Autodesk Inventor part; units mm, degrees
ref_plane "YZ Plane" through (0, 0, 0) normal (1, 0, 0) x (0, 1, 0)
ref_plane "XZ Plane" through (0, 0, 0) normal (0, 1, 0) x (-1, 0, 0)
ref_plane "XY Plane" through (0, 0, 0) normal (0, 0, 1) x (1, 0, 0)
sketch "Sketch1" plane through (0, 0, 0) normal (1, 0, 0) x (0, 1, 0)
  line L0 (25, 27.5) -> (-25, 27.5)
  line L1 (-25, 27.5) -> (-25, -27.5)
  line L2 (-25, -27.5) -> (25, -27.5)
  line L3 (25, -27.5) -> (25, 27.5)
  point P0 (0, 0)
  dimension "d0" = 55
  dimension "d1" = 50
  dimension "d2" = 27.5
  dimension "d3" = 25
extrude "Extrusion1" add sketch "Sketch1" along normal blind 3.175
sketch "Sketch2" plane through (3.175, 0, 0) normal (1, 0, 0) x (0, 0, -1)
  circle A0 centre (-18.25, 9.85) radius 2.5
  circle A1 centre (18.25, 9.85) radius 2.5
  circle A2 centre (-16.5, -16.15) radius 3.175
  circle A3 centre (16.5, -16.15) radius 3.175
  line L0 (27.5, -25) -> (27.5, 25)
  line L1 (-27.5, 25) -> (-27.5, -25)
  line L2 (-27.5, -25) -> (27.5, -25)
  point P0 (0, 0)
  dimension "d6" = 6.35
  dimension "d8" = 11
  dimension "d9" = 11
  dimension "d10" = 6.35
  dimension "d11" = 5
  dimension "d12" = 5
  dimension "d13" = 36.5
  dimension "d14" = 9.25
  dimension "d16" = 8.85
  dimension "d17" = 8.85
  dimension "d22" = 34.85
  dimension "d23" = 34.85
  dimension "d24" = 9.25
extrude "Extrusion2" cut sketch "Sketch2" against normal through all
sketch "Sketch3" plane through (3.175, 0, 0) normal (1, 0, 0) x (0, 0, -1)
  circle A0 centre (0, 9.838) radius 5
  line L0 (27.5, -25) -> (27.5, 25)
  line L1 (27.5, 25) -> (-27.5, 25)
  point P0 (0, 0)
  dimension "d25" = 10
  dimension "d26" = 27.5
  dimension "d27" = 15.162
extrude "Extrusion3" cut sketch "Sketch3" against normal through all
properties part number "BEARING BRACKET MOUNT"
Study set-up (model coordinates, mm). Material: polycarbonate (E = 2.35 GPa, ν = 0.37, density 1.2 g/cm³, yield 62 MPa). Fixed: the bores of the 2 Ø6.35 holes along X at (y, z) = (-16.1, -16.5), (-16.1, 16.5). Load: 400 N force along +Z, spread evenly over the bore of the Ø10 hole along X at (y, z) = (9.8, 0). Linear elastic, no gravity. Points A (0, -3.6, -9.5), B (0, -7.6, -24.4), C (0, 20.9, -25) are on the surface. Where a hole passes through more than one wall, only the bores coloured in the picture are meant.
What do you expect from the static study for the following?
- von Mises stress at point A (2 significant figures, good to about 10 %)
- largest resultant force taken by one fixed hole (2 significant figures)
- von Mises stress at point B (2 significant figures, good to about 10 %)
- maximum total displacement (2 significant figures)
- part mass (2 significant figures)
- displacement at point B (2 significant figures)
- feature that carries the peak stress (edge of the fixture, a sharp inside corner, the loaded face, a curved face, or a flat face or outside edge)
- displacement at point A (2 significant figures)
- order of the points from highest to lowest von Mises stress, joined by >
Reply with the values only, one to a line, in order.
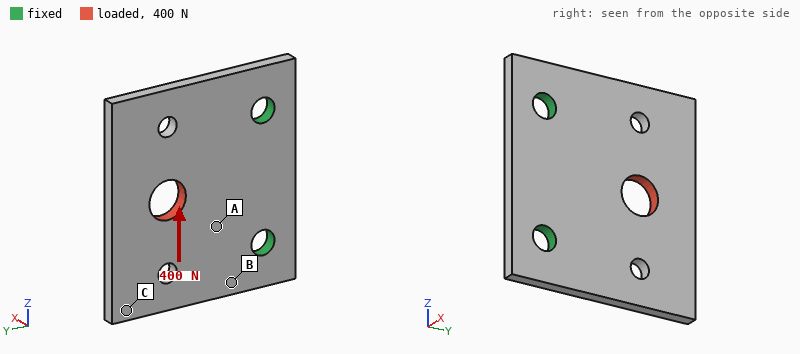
5.5 MPa
330 N
3.1 MPa
0.18 mm
9.8 g
0.053 mm
edge of the fixture
0.050 mm
A > B > C
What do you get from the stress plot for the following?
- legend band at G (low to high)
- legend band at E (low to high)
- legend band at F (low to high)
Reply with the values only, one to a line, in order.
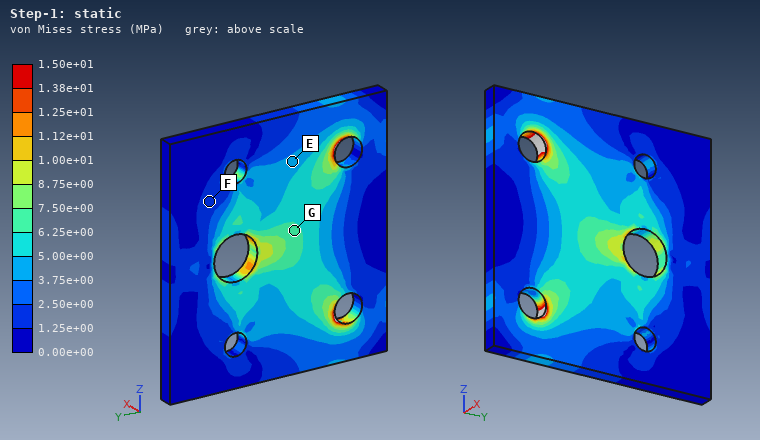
6.25e+00 to 7.50e+00 MPa
3.75e+00 to 5.00e+00 MPa
1.25e+00 to 2.50e+00 MPa
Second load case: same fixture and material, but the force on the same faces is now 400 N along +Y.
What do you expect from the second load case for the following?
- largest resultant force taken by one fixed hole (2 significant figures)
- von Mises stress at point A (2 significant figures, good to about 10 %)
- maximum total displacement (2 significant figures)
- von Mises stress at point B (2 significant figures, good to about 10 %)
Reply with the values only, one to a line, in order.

210 N
3.8 MPa
68 µm
1.0 MPa
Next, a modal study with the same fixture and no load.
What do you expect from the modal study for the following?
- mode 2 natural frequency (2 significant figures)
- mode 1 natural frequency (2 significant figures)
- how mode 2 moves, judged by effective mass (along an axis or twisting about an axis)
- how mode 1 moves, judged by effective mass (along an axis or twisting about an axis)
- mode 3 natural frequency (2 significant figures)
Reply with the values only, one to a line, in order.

840 Hz
460 Hz
twisting about Y
along X
1900 Hz
